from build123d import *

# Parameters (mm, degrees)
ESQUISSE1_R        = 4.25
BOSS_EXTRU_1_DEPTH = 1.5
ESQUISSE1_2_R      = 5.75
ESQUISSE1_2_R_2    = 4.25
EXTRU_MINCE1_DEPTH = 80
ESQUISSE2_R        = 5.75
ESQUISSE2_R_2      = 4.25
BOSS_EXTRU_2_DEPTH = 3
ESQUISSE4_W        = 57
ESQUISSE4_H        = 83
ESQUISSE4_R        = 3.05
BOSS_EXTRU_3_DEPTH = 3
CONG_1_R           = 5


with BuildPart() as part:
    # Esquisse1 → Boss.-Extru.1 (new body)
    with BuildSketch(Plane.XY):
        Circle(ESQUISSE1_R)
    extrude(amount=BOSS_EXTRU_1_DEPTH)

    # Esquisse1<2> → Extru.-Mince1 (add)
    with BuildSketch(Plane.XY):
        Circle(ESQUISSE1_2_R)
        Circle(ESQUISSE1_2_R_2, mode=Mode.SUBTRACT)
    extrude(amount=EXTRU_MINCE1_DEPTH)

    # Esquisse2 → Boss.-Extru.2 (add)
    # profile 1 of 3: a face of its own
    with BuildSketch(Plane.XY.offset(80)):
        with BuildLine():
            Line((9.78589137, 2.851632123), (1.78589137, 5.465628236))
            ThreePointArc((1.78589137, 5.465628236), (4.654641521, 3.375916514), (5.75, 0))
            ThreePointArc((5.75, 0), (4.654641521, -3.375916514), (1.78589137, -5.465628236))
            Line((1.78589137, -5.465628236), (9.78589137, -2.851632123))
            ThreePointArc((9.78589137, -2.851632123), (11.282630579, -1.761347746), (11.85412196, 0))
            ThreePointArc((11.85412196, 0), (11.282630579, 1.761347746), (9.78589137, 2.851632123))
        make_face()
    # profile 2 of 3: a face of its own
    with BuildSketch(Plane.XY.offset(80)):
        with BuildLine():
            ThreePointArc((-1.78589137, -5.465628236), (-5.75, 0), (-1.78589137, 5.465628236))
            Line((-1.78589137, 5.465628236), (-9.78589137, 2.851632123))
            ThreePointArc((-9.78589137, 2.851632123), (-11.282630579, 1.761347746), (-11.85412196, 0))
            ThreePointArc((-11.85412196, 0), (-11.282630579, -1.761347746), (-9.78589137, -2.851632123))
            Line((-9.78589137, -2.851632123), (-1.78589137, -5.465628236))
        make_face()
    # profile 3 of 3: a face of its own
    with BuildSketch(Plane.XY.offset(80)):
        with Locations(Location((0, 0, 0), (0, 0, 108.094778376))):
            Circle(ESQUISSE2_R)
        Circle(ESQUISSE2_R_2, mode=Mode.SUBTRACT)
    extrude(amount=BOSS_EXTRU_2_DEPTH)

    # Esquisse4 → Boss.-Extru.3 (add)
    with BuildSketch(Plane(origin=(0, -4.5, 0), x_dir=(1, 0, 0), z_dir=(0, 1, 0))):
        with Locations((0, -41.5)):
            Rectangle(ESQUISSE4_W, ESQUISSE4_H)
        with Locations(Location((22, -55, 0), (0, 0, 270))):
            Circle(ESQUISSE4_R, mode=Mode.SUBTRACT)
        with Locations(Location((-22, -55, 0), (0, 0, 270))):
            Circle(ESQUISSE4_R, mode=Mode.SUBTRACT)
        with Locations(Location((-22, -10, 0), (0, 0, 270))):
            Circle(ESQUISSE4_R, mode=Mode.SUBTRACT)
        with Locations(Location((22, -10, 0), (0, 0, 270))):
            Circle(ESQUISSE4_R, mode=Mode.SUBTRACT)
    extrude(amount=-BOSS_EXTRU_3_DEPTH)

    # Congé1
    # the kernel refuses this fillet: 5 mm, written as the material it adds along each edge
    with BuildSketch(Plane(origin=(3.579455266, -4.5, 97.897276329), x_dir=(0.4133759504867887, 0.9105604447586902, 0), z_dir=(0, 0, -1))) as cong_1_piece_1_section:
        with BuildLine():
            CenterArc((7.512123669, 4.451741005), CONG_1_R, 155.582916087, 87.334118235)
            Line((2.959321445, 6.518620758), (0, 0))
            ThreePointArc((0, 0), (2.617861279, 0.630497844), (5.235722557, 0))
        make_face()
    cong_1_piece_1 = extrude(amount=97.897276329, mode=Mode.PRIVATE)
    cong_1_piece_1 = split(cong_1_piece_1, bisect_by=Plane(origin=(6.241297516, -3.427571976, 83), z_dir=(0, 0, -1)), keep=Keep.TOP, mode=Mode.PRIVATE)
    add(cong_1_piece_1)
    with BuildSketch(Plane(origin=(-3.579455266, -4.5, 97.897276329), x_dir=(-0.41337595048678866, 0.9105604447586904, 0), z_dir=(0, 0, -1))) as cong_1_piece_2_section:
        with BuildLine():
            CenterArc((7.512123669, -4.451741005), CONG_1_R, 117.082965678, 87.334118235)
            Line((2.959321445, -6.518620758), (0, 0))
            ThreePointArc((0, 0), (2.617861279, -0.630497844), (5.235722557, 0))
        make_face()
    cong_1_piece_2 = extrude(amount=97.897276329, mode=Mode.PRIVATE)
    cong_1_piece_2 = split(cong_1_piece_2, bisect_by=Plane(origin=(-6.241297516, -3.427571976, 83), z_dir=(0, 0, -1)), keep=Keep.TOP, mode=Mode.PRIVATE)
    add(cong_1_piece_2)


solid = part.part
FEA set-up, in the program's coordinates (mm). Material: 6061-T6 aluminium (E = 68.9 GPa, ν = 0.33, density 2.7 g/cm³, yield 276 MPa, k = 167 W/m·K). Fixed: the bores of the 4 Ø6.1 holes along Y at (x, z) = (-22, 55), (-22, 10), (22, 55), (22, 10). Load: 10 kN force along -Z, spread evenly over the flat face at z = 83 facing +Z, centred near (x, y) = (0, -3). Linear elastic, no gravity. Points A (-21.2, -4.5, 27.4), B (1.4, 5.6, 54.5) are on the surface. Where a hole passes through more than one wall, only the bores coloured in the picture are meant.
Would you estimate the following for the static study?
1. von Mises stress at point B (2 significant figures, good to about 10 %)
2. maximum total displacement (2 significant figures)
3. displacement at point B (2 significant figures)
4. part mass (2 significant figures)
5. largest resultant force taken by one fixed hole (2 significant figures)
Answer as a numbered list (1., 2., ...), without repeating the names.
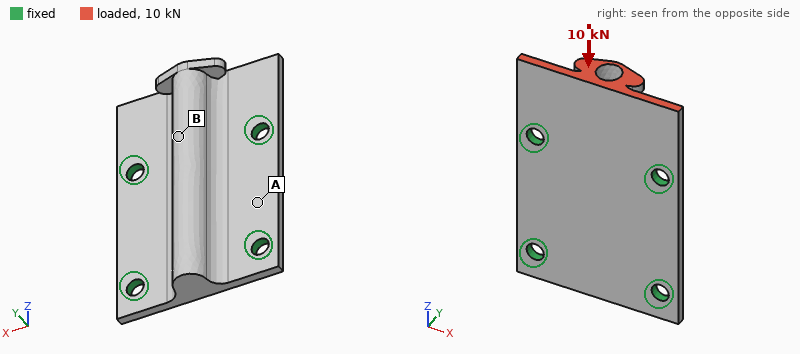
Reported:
1. 98 MPa
2. 0.20 mm
3. 0.049 mm
4. 51 g
5. 3.8 kN
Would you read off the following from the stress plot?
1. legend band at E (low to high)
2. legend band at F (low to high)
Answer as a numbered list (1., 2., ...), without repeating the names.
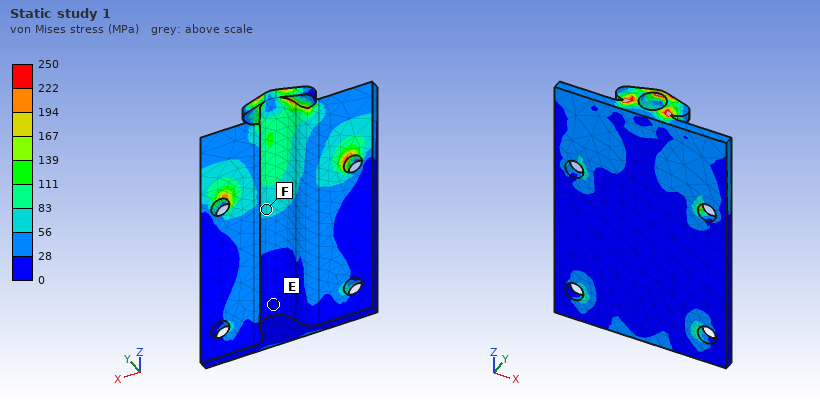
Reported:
1. 0 to 28 MPa
2. 56 to 83 MPa
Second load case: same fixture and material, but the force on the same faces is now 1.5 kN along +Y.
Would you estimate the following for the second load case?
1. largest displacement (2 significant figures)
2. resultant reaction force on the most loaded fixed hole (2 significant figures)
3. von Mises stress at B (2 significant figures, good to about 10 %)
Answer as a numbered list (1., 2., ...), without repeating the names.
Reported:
1. 0.34 mm
2. 1.5 kN
3. 140 MPa
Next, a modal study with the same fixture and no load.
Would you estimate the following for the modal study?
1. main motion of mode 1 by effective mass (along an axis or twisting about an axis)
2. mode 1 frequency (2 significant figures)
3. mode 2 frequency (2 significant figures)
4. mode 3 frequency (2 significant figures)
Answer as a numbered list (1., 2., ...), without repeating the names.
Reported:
1. along Y
2. 4100 Hz
3. 7000 Hz
4. 7000 Hz
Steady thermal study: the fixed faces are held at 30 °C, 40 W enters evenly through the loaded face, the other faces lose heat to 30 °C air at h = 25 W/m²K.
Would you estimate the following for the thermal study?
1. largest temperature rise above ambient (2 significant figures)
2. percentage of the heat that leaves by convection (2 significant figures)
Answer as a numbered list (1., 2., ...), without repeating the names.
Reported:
1. 42 K
2. 7.8 %
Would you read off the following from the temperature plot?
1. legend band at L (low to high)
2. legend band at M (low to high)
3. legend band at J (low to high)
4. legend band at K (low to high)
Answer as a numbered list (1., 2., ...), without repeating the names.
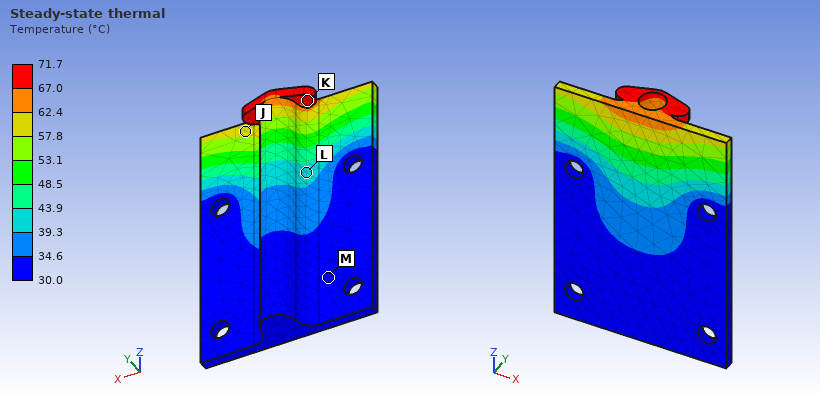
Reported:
1. 39.3 to 43.9 °C
2. 30.0 to 34.6 °C
3. 57.8 to 62.4 °C
4. 67.0 to 71.7 °C
